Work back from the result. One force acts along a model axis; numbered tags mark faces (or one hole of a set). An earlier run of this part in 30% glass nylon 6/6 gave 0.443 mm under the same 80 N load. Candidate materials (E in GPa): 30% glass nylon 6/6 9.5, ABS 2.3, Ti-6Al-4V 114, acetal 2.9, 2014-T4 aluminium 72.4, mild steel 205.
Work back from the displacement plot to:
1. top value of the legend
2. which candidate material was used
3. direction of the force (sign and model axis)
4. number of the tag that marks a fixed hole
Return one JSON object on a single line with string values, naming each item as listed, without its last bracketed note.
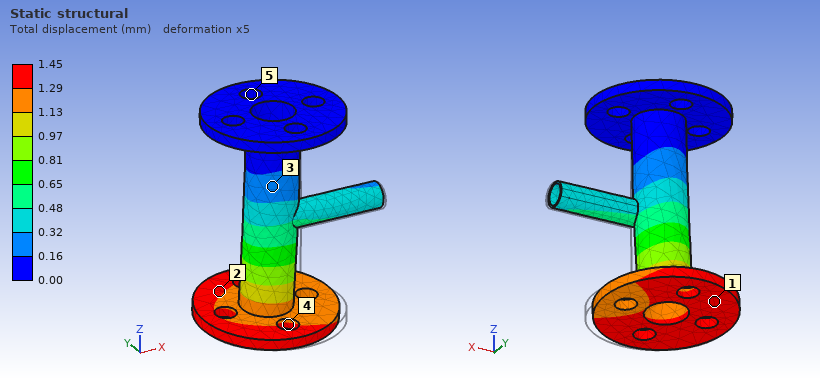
{"top value of the legend": "1.45 mm", "which candidate material was used": "acetal", "direction of the force": "+Y", "number of the tag that marks a fixed hole": "5"}
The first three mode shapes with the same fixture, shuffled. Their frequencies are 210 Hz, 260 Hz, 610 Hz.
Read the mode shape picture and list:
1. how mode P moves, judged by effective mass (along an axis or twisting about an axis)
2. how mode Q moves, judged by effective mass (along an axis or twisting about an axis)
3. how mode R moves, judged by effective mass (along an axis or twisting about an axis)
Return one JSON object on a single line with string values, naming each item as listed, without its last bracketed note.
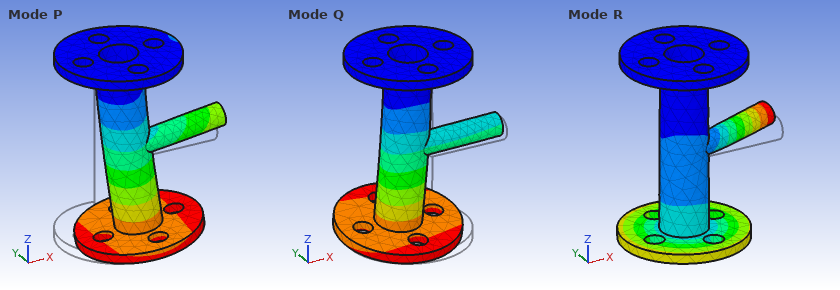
{"how mode P moves, judged by effective mass": "along X", "how mode Q moves, judged by effective mass": "along Y", "how mode R moves, judged by effective mass": "twisting about Z"}
